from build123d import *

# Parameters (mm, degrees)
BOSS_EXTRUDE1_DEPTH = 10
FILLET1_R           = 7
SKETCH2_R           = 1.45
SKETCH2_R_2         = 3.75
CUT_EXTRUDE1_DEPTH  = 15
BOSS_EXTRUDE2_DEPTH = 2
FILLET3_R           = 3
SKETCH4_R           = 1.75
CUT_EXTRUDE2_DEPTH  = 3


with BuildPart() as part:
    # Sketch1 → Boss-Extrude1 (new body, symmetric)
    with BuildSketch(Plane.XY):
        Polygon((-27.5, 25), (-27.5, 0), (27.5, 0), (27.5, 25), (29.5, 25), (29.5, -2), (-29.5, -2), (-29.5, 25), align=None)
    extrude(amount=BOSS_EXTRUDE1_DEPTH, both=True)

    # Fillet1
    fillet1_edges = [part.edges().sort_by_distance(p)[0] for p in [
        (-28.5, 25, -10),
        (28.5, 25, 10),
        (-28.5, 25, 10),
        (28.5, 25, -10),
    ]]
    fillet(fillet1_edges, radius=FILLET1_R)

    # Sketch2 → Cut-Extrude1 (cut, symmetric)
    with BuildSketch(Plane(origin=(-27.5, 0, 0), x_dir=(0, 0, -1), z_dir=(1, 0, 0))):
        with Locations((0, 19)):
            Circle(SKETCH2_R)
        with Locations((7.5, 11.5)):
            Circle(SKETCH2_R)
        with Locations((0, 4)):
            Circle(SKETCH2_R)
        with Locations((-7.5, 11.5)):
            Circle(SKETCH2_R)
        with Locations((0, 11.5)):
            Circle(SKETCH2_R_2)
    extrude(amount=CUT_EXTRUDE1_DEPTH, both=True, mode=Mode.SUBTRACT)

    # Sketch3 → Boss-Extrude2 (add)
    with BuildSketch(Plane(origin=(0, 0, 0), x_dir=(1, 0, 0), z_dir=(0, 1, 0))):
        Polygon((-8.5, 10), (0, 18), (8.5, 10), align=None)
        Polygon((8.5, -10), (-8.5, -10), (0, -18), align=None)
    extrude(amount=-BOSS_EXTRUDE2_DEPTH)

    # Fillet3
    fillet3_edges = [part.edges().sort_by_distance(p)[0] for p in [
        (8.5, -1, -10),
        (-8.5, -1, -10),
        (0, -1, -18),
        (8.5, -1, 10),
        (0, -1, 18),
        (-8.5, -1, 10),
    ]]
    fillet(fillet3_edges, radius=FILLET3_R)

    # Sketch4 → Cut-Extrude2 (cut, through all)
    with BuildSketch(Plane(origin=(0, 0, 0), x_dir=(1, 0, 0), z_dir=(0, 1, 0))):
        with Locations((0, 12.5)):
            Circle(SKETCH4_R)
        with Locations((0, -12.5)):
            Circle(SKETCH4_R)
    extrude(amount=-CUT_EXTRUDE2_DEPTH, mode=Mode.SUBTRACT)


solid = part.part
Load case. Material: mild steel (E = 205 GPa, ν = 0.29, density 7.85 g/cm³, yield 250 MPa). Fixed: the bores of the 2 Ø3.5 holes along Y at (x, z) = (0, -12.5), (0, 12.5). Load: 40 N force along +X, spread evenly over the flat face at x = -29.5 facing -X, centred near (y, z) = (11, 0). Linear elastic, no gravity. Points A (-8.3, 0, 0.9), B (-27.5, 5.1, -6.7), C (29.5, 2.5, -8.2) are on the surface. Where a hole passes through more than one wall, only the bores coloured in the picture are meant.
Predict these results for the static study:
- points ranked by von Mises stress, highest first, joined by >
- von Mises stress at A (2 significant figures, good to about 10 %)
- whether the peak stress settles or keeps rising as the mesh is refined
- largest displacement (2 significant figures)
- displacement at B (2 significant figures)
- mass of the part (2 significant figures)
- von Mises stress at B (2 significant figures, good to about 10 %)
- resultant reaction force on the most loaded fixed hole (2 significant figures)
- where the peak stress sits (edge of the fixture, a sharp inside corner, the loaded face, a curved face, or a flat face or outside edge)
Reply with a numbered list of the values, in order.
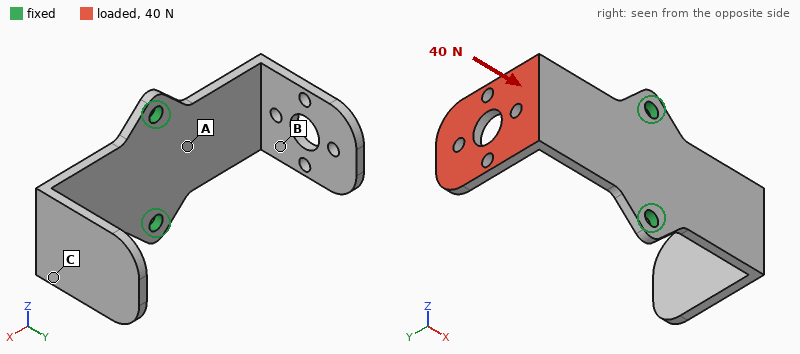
1. A > B > C
2. 32 MPa
3. keeps rising
4. 0.17 mm
5. 0.069 mm
6. 34 g
7. 23 MPa
8. 20 N
9. edge of the fixture
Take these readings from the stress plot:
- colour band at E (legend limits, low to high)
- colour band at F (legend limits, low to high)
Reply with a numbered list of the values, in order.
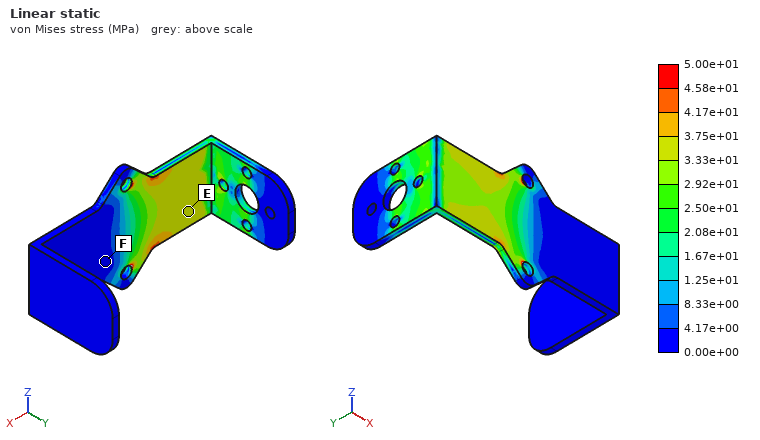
1. 3.33e+01 to 3.75e+01 MPa
2. 0.00e+00 to 4.17e+00 MPa
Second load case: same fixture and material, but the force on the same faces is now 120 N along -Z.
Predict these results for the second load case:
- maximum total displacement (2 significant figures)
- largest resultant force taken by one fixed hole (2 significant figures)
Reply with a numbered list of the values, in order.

1. 0.18 mm
2. 170 N
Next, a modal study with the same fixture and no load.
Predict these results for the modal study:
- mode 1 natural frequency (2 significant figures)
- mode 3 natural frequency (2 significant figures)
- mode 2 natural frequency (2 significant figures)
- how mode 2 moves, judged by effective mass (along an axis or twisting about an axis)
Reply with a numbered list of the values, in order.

1. 760 Hz
2. 1600 Hz
3. 860 Hz
4. along Y
